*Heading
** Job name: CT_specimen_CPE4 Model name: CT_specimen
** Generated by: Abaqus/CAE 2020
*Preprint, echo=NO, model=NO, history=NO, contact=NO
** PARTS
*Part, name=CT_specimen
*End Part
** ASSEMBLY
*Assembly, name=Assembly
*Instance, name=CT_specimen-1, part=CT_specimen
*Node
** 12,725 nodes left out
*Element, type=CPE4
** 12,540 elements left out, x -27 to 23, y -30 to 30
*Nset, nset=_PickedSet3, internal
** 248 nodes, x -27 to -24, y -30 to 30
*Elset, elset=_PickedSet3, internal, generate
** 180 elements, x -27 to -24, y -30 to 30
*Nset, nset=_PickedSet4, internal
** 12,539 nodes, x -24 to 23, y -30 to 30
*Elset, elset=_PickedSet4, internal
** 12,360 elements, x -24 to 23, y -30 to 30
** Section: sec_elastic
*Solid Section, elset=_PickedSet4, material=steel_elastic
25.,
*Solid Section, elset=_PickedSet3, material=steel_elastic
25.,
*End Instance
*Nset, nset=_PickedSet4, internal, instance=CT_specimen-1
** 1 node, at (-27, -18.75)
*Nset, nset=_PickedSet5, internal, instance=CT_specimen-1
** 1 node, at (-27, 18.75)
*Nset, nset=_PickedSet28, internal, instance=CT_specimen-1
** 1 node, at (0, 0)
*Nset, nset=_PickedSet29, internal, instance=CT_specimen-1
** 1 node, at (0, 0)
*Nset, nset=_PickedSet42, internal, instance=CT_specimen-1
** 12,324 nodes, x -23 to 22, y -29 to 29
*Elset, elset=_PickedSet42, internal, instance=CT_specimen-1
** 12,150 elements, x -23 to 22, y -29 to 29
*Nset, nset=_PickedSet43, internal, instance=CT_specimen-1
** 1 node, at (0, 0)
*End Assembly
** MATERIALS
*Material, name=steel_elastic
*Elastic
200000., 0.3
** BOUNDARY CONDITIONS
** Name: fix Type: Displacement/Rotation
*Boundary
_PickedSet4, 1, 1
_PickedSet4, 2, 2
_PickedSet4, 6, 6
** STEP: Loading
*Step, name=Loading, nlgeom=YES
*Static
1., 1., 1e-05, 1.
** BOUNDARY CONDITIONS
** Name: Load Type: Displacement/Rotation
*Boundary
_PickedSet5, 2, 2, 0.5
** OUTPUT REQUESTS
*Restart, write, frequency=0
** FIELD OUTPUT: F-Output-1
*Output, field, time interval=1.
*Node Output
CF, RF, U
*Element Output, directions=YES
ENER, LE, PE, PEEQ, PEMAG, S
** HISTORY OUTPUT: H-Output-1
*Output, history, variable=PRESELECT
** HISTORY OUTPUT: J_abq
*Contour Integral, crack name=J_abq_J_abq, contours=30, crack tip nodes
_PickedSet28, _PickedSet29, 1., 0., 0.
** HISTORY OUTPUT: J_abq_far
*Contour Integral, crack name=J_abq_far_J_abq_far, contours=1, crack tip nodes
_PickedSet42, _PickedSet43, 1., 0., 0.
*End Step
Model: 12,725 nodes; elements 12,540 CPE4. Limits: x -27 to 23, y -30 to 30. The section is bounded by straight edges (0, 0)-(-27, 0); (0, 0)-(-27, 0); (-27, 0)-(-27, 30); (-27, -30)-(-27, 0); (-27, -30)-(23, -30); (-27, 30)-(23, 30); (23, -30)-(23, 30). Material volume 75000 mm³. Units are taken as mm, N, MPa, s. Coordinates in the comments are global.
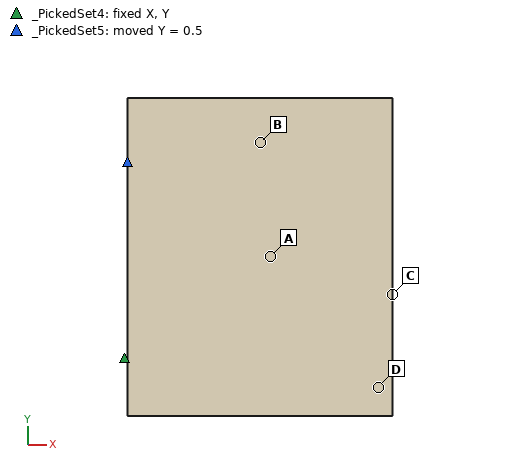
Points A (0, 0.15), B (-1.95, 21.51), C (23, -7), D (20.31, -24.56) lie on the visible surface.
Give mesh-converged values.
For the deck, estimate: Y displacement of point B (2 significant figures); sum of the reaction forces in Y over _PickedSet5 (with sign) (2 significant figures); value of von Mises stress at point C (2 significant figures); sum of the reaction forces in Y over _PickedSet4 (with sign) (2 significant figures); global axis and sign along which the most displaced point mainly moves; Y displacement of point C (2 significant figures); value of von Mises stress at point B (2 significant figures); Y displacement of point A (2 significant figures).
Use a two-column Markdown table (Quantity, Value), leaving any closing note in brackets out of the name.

| Quantity | Value |
|---|---|
| Y displacement of point B | 0.30 mm |
| sum of the reaction forces in Y over _PickedSet5 (with sign) | 56000 N |
| value of von Mises stress at point C | 510 MPa |
| sum of the reaction forces in Y over _PickedSet4 (with sign) | -56000 N |
| global axis and sign along which the most displaced point mainly moves | +Y |
| Y displacement of point C | 0.27 mm |
| value of von Mises stress at point B | 170 MPa |
| Y displacement of point A | 0.25 mm |
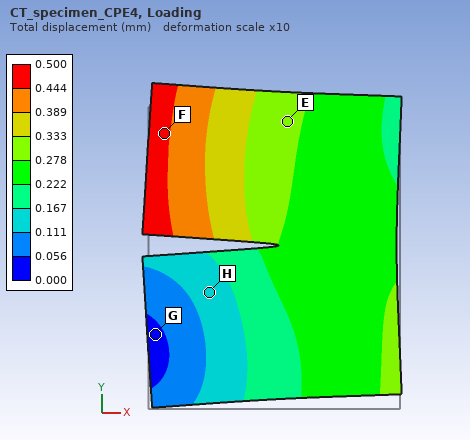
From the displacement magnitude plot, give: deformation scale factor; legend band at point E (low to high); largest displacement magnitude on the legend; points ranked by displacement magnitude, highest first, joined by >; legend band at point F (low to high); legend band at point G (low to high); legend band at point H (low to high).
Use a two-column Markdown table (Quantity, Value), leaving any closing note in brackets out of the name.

| Quantity | Value |
|---|---|
| deformation scale factor | 10 |
| legend band at point E | 0.278 to 0.333 mm |
| largest displacement magnitude on the legend | 0.500 mm |
| points ranked by displacement magnitude, highest first, joined by > | F > E > H > G |
| legend band at point F | 0.444 to 0.500 mm |
| legend band at point G | 0.000 to 0.056 mm |
| legend band at point H | 0.111 to 0.167 mm |
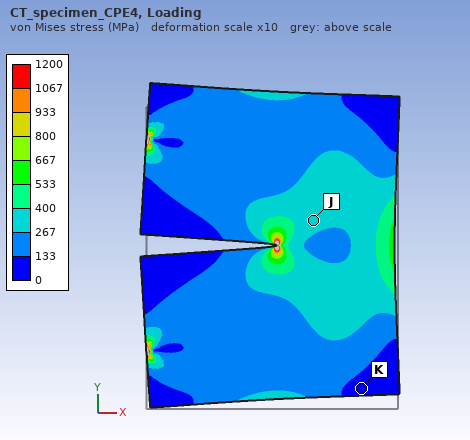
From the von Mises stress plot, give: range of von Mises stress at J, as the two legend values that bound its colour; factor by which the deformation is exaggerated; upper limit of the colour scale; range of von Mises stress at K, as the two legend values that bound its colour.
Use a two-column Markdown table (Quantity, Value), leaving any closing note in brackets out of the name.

| Quantity | Value |
|---|---|
| range of von Mises stress at J, as the two legend values that bound its colour | 267 to 400 MPa |
| factor by which the deformation is exaggerated | 10 |
| upper limit of the colour scale | 1200 MPa |
| range of von Mises stress at K, as the two legend values that bound its colour | 0 to 133 MPa |
